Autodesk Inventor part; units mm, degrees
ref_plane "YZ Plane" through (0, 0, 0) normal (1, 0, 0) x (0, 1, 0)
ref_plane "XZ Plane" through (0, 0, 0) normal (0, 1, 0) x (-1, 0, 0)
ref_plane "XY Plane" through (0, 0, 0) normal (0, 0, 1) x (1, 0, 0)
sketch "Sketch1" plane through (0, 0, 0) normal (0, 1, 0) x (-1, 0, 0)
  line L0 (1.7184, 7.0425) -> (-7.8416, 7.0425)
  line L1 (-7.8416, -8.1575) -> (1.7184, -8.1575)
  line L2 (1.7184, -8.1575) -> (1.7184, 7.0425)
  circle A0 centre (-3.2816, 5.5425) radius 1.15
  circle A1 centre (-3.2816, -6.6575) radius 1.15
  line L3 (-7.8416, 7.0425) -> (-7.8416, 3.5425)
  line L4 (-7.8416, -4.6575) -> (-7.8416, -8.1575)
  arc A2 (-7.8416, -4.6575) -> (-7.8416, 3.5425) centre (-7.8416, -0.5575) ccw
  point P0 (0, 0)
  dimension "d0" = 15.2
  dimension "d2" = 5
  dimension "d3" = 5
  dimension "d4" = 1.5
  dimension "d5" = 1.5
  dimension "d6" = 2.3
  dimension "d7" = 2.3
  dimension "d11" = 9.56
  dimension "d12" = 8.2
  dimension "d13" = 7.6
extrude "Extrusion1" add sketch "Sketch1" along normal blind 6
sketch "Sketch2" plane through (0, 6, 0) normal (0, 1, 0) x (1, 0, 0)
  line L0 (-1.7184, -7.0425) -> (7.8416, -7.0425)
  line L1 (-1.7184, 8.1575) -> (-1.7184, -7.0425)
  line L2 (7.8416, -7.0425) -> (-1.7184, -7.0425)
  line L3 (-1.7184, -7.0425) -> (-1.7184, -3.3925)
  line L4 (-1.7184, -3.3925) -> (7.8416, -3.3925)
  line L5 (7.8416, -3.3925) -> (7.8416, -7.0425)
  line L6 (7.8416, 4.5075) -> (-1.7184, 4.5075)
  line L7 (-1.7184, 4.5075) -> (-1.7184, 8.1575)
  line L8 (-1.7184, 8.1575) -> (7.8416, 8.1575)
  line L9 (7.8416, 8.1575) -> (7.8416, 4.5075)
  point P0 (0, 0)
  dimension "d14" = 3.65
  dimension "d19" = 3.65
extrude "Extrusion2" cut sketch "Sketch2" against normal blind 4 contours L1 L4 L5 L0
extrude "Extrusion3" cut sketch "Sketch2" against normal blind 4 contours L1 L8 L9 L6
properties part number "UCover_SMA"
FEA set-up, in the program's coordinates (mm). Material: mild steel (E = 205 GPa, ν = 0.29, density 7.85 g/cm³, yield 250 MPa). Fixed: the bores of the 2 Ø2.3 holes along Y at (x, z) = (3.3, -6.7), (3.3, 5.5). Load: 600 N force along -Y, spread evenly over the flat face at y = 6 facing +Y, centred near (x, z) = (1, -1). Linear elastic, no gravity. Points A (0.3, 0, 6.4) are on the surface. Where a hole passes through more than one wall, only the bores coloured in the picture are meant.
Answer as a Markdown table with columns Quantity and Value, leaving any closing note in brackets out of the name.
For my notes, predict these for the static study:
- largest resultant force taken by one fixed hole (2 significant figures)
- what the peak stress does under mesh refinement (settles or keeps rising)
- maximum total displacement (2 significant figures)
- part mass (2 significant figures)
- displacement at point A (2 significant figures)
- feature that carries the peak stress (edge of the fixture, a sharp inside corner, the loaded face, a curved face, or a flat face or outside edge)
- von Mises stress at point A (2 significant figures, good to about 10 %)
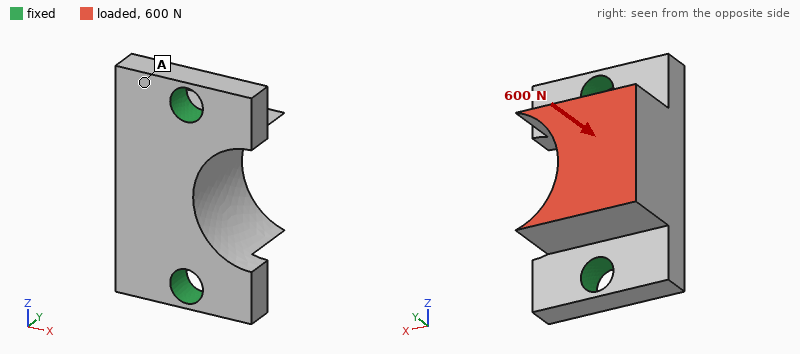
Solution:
| Quantity | Value |
|---|---|
| largest resultant force taken by one fixed hole | 310 N |
| what the peak stress does under mesh refinement | keeps rising |
| maximum total displacement | 6.2 µm |
| part mass | 3.3 g |
| displacement at point A | 1.3 µm |
| feature that carries the peak stress | edge of the fixture |
| von Mises stress at point A | 35 MPa |
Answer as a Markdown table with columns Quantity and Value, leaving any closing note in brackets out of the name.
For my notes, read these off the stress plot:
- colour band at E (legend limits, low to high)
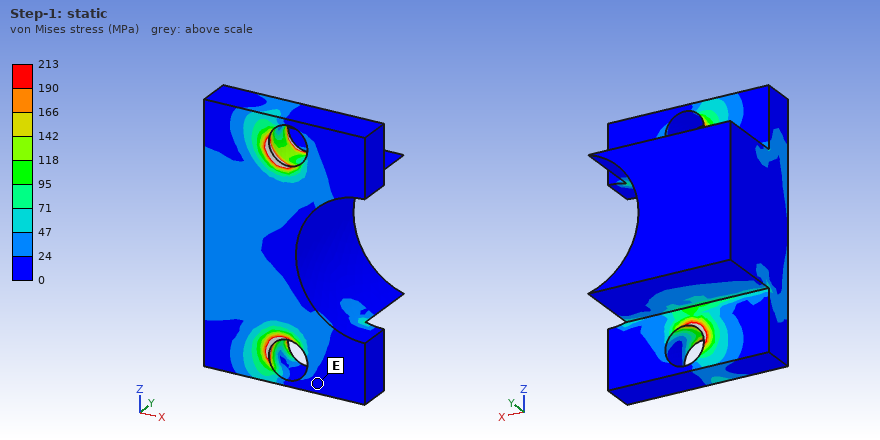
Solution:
| Quantity | Value |
|---|---|
| colour band at E | 0 to 24 MPa |
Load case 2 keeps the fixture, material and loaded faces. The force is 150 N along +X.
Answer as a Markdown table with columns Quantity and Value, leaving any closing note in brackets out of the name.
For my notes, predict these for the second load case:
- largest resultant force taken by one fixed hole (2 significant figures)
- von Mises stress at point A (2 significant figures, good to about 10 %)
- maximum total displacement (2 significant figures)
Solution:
| Quantity | Value |
|---|---|
| largest resultant force taken by one fixed hole | 82 N |
| von Mises stress at point A | 21 MPa |
| maximum total displacement | 4.1 µm |
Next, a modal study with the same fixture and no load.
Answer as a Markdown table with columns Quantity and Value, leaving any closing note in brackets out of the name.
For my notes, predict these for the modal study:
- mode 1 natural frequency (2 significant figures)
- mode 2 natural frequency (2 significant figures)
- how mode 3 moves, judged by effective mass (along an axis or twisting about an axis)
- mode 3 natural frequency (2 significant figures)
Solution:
| Quantity | Value |
|---|---|
| mode 1 natural frequency | 31 kHz |
| mode 2 natural frequency | 67 kHz |
| how mode 3 moves, judged by effective mass | along Z |
| mode 3 natural frequency | 72 kHz |
